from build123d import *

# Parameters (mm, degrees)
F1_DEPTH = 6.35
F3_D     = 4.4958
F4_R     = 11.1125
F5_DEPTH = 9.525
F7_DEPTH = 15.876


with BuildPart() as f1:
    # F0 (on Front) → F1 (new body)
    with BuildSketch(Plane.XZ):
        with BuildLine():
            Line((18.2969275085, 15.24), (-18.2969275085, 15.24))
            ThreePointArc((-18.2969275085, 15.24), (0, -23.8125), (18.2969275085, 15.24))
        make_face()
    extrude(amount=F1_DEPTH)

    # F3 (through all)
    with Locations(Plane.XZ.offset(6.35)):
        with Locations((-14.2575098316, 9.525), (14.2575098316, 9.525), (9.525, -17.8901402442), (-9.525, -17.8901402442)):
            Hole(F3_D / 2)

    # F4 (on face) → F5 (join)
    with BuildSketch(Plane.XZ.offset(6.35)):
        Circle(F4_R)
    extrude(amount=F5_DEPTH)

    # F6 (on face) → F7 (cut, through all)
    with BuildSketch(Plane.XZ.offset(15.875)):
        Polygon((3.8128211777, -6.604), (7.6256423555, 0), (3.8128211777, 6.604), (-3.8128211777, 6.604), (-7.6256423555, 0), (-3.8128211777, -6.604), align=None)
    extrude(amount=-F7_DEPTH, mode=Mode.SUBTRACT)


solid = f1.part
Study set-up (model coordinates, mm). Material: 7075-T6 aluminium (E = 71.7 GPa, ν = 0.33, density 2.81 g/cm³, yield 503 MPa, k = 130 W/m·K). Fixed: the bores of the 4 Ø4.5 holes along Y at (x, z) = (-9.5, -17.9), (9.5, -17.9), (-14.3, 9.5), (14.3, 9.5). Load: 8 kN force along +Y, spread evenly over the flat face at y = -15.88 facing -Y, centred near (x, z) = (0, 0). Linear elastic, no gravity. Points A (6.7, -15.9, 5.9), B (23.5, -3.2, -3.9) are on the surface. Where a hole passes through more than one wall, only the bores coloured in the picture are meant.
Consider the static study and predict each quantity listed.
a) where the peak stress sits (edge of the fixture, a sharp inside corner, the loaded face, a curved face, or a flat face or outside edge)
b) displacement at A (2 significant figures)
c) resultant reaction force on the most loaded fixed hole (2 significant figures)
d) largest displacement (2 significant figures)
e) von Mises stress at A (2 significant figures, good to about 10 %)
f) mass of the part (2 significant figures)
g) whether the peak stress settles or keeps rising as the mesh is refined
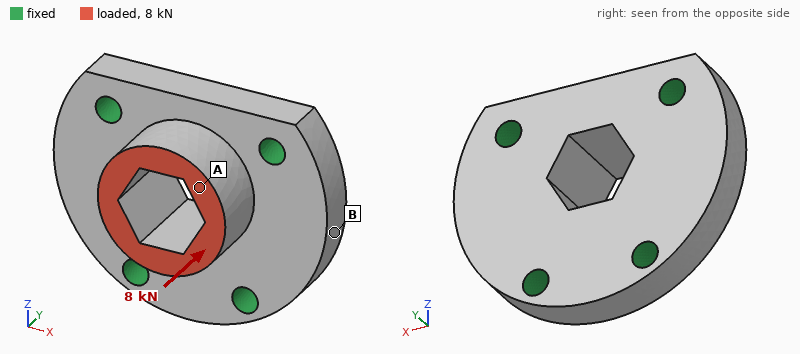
edge of the fixture
19 µm
2.7 kN
22 µm
37 MPa
30 g
keeps rising
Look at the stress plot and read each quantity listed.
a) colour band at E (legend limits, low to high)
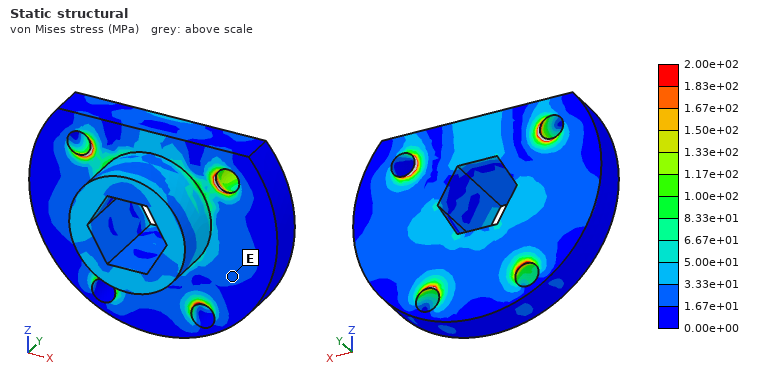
1.67e+01 to 3.33e+01 MPa
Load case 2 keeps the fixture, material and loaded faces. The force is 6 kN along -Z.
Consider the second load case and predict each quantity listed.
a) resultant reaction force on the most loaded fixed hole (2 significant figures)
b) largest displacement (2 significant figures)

2.2 kN
58 µm
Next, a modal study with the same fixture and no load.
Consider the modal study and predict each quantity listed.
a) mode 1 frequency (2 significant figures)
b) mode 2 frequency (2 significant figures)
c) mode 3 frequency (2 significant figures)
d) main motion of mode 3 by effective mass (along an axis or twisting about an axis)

27 kHz
27 kHz
30 kHz
along Y
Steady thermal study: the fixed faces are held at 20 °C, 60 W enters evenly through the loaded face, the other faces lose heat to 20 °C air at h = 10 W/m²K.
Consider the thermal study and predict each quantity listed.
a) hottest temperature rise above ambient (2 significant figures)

32 K
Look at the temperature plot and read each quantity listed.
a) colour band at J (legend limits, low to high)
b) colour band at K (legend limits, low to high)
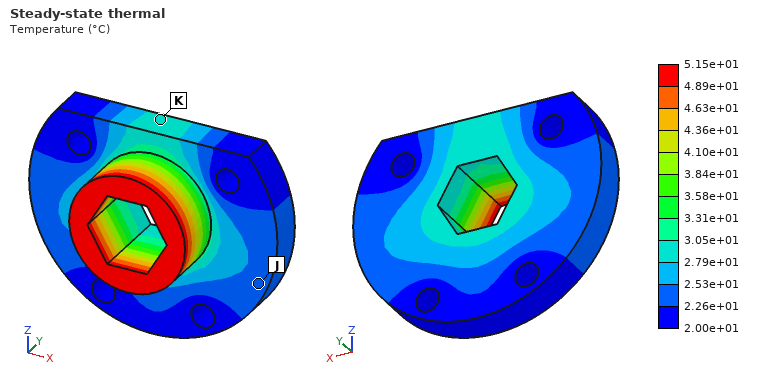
2.26e+01 to 2.53e+01 °C
2.79e+01 to 3.05e+01 °C
